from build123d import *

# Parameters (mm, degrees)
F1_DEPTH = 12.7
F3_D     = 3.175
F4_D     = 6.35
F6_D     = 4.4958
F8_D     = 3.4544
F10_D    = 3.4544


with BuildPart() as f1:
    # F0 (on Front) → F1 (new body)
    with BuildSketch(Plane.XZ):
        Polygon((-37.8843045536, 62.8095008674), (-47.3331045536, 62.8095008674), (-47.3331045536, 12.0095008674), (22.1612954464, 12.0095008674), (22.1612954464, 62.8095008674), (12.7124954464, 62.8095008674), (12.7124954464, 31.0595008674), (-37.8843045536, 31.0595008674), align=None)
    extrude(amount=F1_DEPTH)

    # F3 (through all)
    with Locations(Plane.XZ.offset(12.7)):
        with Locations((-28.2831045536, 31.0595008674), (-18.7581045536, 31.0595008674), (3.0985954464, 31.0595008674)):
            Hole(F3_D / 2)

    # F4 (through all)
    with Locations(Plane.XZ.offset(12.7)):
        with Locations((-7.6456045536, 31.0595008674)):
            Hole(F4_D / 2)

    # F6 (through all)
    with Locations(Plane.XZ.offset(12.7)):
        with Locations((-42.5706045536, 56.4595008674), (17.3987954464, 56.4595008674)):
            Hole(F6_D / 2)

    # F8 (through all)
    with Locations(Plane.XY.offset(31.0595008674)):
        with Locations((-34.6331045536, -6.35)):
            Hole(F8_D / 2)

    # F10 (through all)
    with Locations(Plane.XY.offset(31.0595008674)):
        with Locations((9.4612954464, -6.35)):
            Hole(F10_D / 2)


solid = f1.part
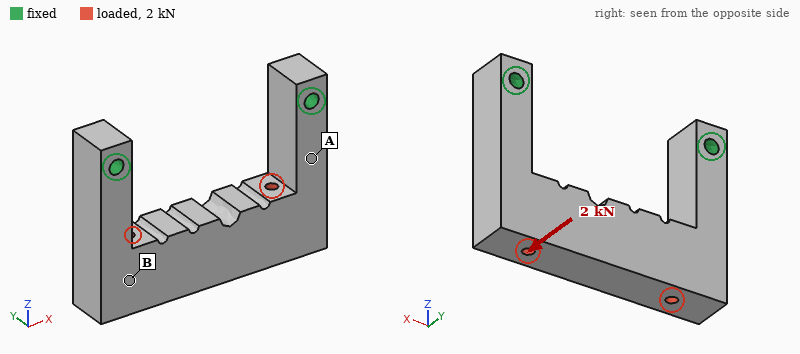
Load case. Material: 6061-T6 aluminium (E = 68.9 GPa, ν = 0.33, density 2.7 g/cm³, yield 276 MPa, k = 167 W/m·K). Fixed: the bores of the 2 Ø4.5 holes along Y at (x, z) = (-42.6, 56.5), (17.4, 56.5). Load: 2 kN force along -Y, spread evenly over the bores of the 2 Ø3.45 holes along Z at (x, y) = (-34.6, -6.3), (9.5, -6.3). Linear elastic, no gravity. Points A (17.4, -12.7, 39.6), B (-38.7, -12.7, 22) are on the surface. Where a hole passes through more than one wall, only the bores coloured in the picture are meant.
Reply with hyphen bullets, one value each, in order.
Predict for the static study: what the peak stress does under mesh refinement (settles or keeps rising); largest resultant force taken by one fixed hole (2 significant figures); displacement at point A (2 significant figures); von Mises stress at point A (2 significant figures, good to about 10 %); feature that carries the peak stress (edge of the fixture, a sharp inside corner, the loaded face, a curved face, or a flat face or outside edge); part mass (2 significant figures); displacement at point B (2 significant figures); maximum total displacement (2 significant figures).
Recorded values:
- keeps rising
- 1.0 kN
- 0.046 mm
- 72 MPa
- edge of the fixture
- 63 g
- 0.13 mm
- 0.20 mm
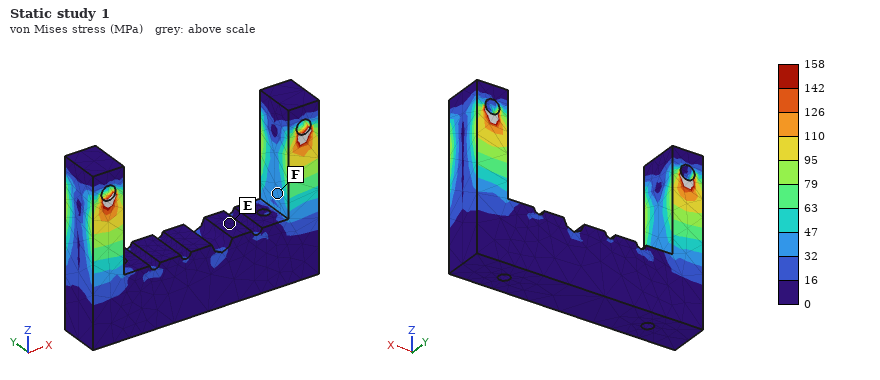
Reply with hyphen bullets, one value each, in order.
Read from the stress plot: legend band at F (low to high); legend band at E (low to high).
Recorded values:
- 32 to 47 MPa
- 0 to 16 MPa
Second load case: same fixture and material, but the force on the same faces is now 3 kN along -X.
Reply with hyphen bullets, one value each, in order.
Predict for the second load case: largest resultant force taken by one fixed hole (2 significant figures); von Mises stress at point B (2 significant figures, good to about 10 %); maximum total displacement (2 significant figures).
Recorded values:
- 1.8 kN
- 20 MPa
- 91 µm
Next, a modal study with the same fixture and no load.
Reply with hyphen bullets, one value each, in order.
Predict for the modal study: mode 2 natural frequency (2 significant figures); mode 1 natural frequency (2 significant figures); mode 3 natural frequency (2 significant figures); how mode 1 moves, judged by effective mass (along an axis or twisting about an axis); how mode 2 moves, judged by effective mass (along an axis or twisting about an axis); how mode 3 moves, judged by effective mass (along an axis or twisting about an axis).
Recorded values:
- 4300 Hz
- 2700 Hz
- 6000 Hz
- along Y
- along X
- twisting about Z
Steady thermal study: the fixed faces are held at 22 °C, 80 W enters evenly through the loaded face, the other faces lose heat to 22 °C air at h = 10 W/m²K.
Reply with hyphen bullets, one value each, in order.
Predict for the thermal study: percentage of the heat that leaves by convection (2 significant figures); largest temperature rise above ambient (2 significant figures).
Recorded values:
- 4.1 %
- 65 K
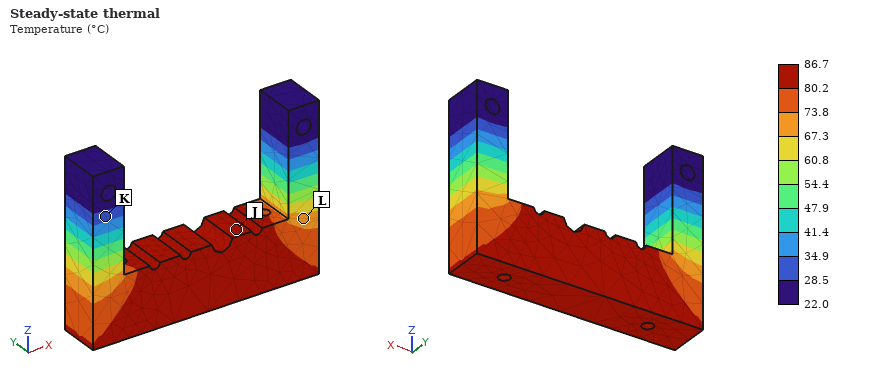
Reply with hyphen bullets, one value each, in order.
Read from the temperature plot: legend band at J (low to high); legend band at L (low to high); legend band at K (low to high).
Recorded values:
- 80.2 to 86.7 °C
- 67.3 to 73.8 °C
- 28.5 to 34.9 °C
